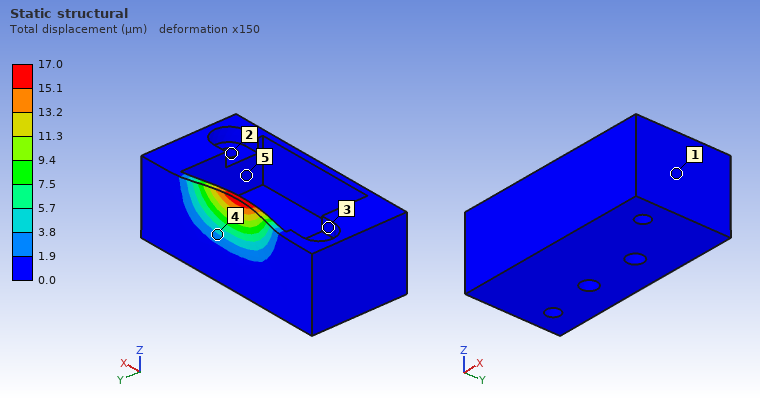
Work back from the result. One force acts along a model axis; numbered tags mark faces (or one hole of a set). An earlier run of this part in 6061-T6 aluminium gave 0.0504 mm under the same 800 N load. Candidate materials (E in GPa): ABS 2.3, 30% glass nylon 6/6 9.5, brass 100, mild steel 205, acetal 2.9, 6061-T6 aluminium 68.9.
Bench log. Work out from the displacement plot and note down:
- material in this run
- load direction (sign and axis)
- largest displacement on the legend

mild steel
-Y
17.0 µm
